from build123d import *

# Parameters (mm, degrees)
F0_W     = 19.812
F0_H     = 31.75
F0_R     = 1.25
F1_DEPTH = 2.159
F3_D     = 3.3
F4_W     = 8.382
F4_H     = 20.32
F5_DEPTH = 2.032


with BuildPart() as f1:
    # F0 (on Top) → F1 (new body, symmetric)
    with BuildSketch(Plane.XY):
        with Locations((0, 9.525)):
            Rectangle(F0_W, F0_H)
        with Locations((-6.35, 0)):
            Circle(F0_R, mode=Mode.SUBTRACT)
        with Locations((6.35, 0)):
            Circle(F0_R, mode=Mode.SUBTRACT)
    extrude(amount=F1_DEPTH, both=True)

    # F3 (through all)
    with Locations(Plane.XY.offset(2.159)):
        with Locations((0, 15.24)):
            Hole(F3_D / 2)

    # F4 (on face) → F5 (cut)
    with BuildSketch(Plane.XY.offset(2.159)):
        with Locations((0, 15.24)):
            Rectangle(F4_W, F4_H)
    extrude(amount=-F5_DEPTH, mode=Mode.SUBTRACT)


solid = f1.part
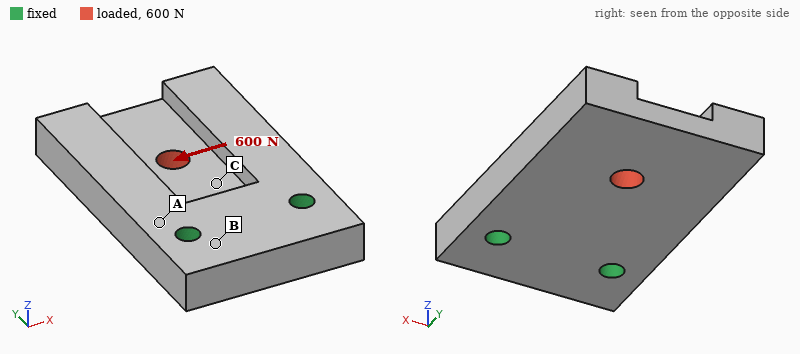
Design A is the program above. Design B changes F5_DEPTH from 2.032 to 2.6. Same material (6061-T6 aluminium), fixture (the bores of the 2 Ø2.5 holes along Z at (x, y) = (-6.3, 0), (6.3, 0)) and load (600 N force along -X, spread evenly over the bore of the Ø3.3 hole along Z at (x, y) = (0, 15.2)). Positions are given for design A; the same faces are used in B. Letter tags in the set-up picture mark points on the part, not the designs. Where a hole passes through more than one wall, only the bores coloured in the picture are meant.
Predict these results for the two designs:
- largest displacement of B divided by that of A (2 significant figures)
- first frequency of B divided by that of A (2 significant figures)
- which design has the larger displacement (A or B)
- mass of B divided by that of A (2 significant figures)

1.1
1.0
B
0.96
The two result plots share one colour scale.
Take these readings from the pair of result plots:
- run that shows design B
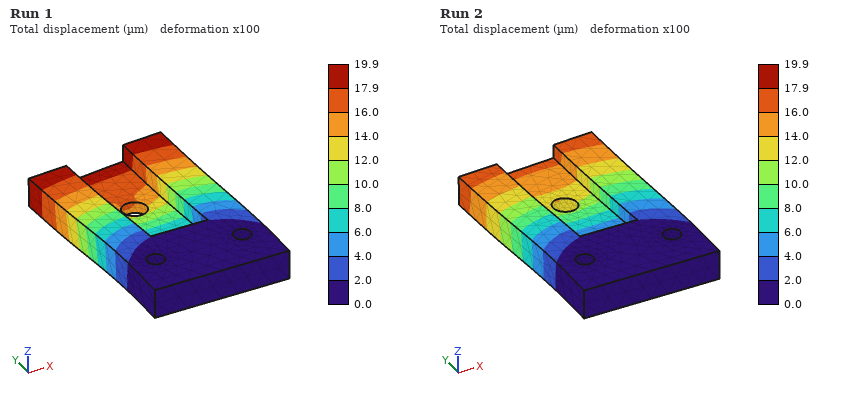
Run 1
